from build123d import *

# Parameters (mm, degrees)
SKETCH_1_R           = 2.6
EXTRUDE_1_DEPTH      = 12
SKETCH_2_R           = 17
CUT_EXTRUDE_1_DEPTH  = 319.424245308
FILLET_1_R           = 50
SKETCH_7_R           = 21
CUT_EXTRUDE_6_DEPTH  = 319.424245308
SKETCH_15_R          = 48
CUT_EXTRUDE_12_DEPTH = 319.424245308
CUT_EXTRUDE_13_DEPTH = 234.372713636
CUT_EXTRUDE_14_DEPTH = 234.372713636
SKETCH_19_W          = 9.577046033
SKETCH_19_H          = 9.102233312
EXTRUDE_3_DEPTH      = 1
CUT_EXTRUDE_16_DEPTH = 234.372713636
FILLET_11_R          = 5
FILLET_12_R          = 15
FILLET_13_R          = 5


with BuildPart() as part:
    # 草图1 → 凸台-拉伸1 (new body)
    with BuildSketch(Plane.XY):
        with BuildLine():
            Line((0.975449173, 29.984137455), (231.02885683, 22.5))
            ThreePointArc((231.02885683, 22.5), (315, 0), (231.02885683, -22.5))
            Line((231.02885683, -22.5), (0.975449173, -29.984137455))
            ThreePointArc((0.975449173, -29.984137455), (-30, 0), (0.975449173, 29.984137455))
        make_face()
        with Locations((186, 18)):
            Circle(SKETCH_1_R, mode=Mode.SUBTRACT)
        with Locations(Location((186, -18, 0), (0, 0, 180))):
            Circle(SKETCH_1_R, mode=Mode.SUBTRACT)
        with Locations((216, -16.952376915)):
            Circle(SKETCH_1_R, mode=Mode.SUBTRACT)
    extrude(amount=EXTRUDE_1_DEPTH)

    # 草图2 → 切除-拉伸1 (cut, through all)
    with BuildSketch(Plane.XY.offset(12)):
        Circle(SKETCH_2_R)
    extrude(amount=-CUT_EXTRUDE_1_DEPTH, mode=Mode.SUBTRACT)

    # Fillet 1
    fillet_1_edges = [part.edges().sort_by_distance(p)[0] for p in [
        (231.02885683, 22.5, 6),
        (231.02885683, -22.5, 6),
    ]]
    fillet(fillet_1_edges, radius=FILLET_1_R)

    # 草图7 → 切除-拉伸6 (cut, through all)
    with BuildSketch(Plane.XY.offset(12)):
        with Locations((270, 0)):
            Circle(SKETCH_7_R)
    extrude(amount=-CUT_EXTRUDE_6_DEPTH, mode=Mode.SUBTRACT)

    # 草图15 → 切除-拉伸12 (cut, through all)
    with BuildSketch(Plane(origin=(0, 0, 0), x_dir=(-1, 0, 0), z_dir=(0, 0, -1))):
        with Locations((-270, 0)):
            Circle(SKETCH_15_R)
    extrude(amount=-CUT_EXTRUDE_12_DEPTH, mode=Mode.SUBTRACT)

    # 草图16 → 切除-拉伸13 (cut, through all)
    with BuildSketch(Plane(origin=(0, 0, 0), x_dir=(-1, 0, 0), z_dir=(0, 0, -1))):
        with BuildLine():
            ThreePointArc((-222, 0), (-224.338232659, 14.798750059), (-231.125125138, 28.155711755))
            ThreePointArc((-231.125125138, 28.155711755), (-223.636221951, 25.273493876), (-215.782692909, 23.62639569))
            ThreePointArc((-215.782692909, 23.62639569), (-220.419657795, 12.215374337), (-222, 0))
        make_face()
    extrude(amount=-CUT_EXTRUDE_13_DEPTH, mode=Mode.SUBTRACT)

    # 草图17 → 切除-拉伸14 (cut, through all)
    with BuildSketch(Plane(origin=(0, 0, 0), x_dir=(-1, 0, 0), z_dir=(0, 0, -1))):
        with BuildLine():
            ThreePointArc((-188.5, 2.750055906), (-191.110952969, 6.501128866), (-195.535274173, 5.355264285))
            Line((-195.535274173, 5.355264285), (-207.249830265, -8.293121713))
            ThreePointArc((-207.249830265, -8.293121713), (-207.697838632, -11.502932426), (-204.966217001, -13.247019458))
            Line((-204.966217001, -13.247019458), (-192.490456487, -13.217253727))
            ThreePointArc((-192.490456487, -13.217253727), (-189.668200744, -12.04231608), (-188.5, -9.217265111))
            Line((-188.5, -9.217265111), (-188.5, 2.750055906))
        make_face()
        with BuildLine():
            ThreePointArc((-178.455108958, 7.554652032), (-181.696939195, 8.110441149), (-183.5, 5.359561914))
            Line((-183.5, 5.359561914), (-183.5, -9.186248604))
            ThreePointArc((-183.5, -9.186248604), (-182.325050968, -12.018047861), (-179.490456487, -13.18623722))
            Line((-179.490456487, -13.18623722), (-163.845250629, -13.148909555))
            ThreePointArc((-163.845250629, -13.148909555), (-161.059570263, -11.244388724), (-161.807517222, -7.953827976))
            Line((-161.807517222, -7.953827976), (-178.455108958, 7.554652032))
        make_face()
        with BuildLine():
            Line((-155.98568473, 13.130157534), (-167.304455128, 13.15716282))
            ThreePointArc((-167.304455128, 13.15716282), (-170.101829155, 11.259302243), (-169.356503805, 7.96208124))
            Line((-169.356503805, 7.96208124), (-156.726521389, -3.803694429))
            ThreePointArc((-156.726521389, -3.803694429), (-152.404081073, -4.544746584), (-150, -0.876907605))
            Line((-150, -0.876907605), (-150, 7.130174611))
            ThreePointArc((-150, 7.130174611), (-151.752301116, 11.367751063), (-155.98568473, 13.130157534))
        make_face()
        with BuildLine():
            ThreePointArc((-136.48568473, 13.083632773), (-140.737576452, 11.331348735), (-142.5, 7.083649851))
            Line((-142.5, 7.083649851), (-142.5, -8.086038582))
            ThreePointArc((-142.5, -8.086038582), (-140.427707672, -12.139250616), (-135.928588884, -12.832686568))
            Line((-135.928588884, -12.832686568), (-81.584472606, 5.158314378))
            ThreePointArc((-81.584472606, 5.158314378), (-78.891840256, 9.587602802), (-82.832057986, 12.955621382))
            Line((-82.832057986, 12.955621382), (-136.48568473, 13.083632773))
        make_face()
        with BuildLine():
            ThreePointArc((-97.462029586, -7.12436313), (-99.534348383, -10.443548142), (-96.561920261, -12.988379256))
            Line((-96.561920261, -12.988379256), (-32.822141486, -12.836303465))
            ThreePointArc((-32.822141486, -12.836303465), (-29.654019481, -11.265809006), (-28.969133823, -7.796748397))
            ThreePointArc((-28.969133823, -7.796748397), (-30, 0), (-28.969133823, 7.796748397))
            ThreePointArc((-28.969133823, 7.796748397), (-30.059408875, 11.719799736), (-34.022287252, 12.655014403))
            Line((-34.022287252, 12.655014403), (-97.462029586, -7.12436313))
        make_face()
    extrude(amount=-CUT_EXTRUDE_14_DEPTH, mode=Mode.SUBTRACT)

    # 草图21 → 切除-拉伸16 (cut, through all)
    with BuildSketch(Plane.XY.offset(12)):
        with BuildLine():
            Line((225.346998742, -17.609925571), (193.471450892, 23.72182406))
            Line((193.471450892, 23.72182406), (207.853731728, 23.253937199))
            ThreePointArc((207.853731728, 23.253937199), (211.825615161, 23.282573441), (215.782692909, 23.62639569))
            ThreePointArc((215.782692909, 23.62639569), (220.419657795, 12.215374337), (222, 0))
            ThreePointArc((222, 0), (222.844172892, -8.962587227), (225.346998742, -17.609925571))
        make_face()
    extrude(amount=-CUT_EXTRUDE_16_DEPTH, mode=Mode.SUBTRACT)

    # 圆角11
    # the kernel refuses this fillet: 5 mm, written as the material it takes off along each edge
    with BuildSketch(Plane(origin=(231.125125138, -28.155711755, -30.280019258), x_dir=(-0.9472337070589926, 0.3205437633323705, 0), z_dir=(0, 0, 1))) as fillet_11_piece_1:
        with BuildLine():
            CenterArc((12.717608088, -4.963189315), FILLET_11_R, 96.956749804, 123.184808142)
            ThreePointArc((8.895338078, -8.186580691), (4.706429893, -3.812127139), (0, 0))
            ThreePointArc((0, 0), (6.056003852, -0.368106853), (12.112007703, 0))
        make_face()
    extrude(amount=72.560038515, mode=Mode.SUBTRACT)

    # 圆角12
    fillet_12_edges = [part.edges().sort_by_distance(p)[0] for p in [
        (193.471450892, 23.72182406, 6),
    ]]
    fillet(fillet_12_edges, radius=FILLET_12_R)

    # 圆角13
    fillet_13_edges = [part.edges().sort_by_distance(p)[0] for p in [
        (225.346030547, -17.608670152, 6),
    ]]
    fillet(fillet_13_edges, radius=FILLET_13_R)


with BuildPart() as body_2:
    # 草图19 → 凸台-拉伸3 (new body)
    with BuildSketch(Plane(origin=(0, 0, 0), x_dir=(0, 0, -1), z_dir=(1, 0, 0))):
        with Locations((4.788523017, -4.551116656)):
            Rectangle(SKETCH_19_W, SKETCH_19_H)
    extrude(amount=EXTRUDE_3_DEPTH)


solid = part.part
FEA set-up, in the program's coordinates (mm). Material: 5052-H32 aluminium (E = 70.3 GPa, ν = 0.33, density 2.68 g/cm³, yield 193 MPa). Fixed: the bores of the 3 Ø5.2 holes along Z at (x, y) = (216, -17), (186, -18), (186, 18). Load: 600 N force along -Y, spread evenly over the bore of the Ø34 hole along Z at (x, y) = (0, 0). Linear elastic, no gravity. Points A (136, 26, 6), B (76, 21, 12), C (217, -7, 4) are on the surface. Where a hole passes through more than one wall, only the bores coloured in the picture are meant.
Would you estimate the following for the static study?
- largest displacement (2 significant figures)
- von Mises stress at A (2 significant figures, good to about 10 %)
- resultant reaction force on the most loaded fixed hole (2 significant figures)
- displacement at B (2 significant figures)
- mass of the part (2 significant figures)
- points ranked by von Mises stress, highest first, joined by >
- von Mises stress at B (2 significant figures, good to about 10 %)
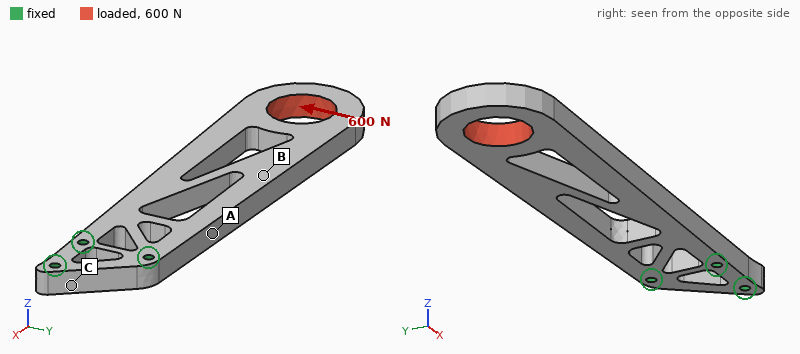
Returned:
0.27 mm
25 MPa
2.9 kN
0.11 mm
280 g
A > B > C
10 MPa
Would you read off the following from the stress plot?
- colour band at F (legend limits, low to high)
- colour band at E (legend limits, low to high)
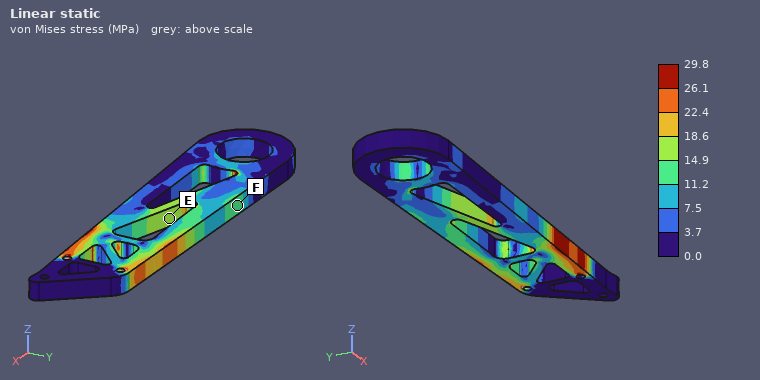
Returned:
11.2 to 14.9 MPa
14.9 to 18.6 MPa
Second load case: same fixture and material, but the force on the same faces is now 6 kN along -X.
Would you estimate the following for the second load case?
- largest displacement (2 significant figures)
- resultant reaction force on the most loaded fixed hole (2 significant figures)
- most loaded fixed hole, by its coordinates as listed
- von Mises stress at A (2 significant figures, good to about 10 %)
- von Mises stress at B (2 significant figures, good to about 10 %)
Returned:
55 µm
3.1 kN
(186, 18)
22 MPa
16 MPa
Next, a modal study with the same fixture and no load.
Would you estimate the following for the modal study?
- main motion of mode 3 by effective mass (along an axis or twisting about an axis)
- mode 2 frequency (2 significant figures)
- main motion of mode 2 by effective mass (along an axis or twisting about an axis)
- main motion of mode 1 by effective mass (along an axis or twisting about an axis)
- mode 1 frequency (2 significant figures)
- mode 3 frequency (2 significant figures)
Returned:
twisting about X
800 Hz
along Y
along Z
190 Hz
1000 Hz
